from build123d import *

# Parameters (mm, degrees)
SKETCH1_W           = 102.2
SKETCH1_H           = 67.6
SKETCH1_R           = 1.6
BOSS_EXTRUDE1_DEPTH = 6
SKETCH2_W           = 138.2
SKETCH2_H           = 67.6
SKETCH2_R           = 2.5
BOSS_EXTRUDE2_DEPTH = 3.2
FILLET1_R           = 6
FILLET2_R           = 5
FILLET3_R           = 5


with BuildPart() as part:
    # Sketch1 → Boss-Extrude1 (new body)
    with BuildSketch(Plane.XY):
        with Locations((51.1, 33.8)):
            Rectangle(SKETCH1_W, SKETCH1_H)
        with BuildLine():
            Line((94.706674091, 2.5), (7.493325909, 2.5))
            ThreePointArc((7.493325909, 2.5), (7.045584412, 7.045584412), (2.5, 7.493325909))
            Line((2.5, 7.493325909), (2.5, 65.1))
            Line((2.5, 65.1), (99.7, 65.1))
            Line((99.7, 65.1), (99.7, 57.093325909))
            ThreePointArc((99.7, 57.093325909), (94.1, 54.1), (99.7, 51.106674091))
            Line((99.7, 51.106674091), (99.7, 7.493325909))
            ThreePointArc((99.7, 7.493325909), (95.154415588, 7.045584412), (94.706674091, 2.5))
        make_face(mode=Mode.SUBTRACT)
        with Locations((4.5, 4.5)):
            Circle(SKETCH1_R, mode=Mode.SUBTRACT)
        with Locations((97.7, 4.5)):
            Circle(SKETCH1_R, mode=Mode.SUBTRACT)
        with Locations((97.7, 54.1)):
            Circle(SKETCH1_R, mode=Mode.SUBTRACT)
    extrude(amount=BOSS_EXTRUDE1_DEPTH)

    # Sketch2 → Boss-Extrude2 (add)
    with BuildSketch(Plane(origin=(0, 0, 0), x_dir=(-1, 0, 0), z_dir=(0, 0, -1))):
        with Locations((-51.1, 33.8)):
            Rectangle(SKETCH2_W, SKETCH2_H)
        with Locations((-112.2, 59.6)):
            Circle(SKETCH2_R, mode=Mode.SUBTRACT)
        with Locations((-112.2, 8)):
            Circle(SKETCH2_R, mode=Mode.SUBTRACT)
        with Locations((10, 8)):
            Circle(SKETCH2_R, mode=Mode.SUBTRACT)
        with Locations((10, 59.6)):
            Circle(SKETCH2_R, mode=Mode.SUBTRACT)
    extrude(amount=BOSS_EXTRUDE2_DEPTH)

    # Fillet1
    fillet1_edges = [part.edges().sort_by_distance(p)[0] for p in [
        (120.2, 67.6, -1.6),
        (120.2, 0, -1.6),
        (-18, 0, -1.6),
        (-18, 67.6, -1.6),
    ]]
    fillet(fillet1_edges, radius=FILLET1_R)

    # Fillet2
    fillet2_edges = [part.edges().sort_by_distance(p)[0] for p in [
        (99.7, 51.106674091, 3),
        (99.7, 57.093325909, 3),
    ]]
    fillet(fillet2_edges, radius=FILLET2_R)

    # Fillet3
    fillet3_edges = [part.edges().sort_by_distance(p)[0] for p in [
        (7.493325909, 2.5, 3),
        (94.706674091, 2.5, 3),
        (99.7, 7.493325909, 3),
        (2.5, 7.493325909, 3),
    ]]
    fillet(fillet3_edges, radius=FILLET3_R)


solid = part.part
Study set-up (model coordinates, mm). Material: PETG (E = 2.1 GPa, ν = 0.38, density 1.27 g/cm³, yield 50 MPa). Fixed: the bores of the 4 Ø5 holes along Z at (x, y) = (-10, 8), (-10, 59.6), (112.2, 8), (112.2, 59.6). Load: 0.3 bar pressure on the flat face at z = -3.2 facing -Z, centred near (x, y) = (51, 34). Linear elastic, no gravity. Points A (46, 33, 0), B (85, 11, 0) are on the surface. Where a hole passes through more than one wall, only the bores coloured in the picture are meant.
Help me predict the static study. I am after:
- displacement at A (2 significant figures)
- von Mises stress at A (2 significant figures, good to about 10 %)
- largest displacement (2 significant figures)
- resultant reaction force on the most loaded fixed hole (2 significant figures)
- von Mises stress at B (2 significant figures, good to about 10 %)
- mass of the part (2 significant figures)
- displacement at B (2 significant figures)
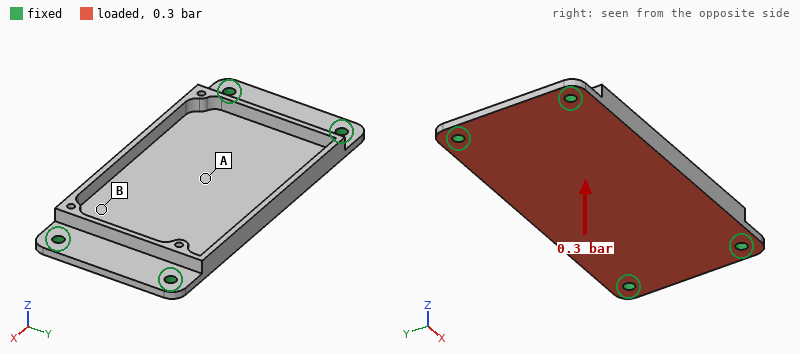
1.6 mm
5.4 MPa
1.6 mm
94 N
2.3 MPa
44 g
0.80 mm
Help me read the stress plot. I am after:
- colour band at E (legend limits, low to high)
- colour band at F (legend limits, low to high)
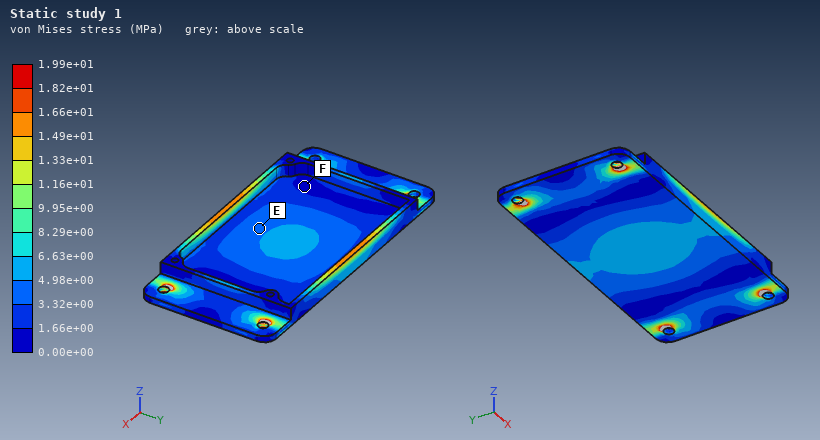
3.32e+00 to 4.98e+00 MPa
0.00e+00 to 1.66e+00 MPa
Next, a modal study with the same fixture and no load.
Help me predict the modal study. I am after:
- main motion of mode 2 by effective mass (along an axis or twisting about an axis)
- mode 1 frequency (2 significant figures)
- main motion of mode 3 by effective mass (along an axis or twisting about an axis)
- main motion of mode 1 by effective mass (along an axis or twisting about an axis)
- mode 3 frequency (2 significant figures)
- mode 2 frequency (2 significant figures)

twisting about X
370 Hz
twisting about Y
along Z
1000 Hz
560 Hz
